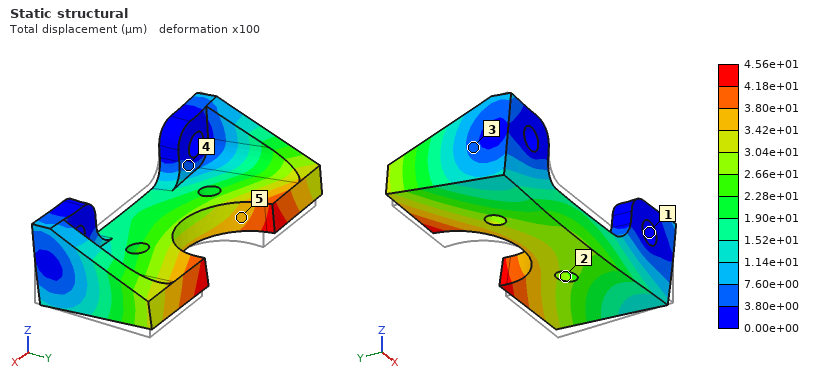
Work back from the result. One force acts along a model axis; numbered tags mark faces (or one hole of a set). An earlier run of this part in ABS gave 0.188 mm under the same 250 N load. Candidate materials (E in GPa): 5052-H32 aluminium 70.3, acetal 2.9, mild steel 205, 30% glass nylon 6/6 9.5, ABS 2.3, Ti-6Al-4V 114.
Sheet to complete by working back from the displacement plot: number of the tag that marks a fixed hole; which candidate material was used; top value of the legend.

1
30% glass nylon 6/6
4.56e+01 µm
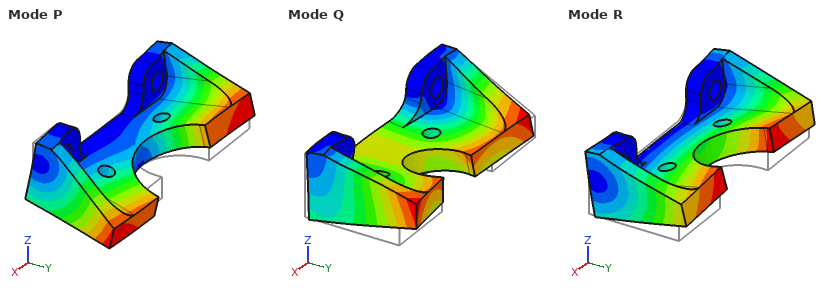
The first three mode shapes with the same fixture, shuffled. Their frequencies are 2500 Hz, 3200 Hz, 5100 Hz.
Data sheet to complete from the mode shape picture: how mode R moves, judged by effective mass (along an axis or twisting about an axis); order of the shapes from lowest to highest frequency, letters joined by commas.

along Z
R, P, Q
